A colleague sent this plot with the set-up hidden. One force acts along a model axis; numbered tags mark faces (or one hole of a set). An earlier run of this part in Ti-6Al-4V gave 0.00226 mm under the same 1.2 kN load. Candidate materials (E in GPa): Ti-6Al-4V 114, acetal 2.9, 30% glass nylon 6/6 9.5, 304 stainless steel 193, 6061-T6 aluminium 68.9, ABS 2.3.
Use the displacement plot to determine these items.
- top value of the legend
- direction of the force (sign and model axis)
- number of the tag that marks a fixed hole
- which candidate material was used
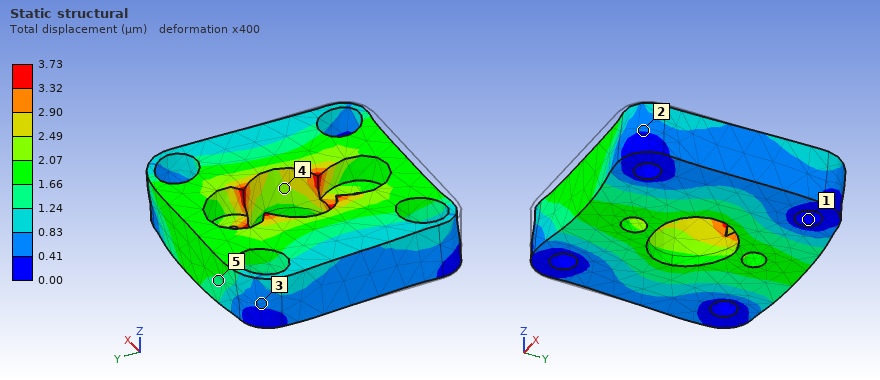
3.73 µm
+Y
1
6061-T6 aluminium
